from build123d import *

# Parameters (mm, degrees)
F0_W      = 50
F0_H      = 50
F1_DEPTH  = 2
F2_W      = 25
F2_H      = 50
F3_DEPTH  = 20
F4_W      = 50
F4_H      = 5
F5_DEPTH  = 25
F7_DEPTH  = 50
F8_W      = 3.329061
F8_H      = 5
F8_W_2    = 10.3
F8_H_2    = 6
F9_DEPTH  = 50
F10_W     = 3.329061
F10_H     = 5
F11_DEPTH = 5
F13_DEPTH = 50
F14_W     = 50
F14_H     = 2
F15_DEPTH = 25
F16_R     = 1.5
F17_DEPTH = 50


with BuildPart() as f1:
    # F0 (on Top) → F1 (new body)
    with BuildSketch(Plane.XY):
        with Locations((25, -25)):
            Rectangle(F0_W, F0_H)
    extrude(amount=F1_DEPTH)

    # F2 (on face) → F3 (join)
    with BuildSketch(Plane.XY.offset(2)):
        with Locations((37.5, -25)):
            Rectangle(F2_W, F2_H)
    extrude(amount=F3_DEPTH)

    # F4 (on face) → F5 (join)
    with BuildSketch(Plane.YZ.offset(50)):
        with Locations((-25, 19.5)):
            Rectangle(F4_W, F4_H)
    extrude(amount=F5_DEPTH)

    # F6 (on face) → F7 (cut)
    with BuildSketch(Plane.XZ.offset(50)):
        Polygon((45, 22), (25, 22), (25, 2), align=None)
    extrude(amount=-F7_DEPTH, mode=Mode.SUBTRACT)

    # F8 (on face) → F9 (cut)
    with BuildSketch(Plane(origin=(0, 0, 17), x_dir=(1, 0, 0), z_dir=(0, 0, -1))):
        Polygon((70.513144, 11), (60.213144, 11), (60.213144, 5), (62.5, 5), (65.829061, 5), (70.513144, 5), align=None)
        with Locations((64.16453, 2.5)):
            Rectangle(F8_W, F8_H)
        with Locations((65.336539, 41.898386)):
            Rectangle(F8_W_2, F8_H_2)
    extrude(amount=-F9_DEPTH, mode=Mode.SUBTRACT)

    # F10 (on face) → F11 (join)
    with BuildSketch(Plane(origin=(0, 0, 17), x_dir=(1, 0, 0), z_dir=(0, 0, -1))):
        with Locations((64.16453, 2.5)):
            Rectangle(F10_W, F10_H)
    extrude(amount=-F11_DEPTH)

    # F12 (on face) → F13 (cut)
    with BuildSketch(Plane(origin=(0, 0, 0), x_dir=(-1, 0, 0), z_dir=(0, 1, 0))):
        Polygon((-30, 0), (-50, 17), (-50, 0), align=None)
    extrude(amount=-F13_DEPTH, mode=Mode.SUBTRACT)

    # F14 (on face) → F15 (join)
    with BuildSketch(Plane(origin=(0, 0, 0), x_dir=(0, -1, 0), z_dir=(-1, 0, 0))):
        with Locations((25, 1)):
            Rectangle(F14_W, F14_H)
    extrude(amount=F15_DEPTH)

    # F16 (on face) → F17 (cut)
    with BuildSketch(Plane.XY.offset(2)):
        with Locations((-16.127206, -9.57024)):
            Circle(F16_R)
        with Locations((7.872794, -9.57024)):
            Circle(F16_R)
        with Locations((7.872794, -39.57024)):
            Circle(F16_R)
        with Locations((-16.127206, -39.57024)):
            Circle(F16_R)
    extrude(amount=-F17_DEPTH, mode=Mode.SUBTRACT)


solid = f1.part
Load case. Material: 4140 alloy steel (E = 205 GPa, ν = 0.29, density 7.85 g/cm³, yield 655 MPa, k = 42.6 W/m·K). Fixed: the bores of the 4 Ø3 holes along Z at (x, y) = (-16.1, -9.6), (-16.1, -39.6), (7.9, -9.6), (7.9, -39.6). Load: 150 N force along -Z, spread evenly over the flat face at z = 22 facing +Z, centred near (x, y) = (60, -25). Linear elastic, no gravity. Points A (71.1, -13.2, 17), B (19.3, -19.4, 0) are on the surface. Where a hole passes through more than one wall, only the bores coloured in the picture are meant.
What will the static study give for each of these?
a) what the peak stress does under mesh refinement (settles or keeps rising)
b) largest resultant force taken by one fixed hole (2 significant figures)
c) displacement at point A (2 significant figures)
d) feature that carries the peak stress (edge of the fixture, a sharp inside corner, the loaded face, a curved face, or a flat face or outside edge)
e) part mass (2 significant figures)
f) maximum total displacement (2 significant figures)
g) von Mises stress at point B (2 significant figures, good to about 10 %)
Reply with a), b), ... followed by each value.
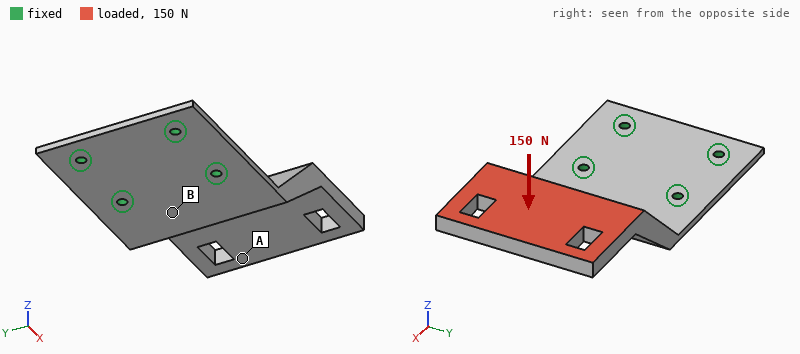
a) keeps rising
b) 130 N
c) 1.00 mm
d) edge of the fixture
e) 150 g
f) 1.1 mm
g) 160 MPa
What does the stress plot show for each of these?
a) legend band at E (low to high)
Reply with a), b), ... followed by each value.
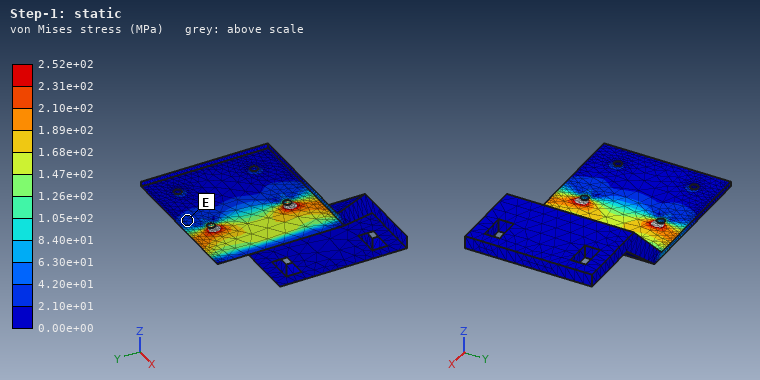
a) 2.10e+01 to 4.20e+01 MPa
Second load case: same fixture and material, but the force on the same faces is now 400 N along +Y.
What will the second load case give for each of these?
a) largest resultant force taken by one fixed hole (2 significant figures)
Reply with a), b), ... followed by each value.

a) 610 N
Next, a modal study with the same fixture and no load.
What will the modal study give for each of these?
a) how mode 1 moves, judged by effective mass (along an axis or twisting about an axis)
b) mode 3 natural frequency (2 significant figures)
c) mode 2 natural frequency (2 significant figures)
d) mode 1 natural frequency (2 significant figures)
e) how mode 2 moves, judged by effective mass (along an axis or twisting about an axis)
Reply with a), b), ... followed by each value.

a) along Z
b) 2600 Hz
c) 1100 Hz
d) 240 Hz
e) along Y
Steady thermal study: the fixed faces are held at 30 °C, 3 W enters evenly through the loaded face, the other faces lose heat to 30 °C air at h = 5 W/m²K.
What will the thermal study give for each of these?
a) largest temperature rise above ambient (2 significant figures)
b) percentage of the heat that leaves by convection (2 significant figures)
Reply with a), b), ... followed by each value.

a) 22 K
b) 18 %
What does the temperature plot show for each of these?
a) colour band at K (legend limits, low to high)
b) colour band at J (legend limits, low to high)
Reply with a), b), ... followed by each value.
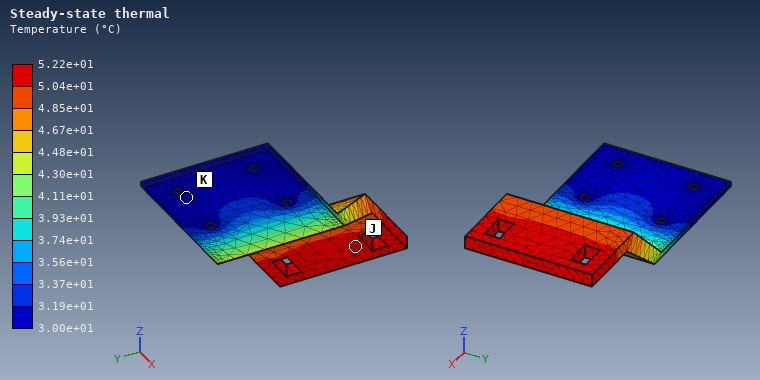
a) 3.00e+01 to 3.19e+01 °C
b) 5.04e+01 to 5.22e+01 °C
